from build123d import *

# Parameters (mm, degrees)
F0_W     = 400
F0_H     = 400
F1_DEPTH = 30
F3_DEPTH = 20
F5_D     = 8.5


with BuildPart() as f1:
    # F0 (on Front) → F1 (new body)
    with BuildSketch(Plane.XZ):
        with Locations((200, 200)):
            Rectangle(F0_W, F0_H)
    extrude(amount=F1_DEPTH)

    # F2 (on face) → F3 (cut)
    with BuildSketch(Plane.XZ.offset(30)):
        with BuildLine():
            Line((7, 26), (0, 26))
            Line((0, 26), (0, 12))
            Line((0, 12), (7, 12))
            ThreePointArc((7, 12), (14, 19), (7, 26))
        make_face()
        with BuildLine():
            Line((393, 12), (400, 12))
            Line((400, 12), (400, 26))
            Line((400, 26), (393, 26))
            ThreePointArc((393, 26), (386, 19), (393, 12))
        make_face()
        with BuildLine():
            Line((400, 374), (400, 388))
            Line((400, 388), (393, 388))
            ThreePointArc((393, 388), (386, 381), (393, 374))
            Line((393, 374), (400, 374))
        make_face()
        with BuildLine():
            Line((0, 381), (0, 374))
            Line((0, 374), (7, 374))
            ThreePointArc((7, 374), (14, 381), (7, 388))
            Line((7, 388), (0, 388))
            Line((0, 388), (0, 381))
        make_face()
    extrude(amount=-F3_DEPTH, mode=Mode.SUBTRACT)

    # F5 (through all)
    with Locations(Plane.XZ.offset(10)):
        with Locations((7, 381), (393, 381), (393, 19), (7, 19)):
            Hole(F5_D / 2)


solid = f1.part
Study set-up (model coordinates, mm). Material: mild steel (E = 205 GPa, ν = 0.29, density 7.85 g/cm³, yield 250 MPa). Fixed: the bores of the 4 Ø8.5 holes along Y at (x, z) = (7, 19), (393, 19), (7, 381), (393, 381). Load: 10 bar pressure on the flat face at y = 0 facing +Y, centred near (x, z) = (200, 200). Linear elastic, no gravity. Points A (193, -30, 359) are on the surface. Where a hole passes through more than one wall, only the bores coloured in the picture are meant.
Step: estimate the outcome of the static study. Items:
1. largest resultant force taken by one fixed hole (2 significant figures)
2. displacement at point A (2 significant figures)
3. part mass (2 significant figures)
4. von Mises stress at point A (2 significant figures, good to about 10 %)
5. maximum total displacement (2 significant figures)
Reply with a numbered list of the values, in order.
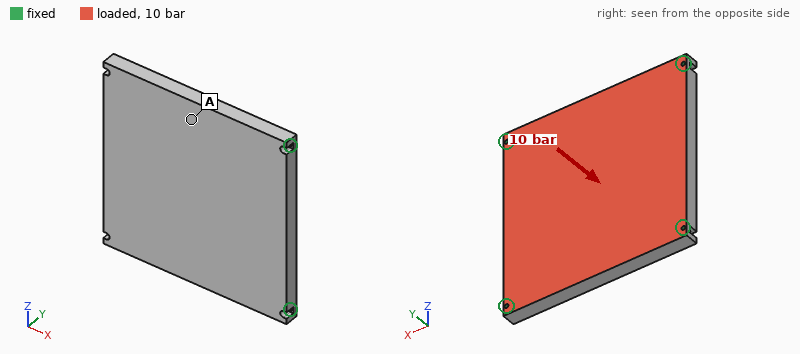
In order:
1. 85 kN
2. 0.50 mm
3. 38 kg
4. 100 MPa
5. 0.66 mm
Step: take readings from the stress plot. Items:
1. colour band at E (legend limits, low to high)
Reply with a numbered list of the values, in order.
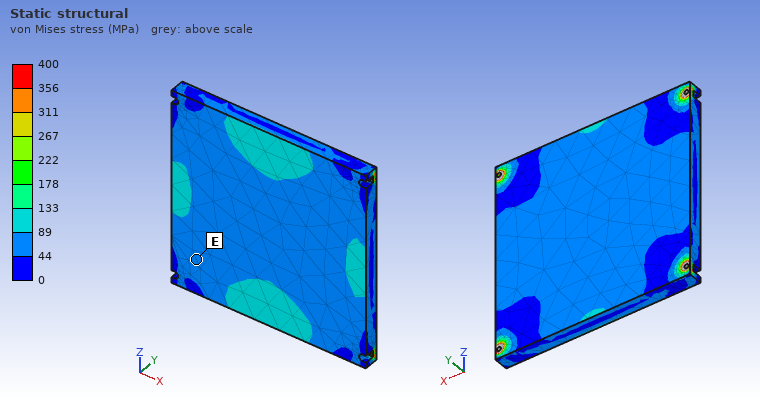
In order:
1. 44 to 89 MPa
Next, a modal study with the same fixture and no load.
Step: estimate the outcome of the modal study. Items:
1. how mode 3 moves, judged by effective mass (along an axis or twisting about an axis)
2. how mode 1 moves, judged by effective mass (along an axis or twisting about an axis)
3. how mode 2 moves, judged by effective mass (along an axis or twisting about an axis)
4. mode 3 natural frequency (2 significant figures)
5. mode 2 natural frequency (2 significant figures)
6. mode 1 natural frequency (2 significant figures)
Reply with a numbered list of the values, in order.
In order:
1. twisting about Z
2. along Y
3. twisting about X
4. 920 Hz
5. 850 Hz
6. 470 Hz
